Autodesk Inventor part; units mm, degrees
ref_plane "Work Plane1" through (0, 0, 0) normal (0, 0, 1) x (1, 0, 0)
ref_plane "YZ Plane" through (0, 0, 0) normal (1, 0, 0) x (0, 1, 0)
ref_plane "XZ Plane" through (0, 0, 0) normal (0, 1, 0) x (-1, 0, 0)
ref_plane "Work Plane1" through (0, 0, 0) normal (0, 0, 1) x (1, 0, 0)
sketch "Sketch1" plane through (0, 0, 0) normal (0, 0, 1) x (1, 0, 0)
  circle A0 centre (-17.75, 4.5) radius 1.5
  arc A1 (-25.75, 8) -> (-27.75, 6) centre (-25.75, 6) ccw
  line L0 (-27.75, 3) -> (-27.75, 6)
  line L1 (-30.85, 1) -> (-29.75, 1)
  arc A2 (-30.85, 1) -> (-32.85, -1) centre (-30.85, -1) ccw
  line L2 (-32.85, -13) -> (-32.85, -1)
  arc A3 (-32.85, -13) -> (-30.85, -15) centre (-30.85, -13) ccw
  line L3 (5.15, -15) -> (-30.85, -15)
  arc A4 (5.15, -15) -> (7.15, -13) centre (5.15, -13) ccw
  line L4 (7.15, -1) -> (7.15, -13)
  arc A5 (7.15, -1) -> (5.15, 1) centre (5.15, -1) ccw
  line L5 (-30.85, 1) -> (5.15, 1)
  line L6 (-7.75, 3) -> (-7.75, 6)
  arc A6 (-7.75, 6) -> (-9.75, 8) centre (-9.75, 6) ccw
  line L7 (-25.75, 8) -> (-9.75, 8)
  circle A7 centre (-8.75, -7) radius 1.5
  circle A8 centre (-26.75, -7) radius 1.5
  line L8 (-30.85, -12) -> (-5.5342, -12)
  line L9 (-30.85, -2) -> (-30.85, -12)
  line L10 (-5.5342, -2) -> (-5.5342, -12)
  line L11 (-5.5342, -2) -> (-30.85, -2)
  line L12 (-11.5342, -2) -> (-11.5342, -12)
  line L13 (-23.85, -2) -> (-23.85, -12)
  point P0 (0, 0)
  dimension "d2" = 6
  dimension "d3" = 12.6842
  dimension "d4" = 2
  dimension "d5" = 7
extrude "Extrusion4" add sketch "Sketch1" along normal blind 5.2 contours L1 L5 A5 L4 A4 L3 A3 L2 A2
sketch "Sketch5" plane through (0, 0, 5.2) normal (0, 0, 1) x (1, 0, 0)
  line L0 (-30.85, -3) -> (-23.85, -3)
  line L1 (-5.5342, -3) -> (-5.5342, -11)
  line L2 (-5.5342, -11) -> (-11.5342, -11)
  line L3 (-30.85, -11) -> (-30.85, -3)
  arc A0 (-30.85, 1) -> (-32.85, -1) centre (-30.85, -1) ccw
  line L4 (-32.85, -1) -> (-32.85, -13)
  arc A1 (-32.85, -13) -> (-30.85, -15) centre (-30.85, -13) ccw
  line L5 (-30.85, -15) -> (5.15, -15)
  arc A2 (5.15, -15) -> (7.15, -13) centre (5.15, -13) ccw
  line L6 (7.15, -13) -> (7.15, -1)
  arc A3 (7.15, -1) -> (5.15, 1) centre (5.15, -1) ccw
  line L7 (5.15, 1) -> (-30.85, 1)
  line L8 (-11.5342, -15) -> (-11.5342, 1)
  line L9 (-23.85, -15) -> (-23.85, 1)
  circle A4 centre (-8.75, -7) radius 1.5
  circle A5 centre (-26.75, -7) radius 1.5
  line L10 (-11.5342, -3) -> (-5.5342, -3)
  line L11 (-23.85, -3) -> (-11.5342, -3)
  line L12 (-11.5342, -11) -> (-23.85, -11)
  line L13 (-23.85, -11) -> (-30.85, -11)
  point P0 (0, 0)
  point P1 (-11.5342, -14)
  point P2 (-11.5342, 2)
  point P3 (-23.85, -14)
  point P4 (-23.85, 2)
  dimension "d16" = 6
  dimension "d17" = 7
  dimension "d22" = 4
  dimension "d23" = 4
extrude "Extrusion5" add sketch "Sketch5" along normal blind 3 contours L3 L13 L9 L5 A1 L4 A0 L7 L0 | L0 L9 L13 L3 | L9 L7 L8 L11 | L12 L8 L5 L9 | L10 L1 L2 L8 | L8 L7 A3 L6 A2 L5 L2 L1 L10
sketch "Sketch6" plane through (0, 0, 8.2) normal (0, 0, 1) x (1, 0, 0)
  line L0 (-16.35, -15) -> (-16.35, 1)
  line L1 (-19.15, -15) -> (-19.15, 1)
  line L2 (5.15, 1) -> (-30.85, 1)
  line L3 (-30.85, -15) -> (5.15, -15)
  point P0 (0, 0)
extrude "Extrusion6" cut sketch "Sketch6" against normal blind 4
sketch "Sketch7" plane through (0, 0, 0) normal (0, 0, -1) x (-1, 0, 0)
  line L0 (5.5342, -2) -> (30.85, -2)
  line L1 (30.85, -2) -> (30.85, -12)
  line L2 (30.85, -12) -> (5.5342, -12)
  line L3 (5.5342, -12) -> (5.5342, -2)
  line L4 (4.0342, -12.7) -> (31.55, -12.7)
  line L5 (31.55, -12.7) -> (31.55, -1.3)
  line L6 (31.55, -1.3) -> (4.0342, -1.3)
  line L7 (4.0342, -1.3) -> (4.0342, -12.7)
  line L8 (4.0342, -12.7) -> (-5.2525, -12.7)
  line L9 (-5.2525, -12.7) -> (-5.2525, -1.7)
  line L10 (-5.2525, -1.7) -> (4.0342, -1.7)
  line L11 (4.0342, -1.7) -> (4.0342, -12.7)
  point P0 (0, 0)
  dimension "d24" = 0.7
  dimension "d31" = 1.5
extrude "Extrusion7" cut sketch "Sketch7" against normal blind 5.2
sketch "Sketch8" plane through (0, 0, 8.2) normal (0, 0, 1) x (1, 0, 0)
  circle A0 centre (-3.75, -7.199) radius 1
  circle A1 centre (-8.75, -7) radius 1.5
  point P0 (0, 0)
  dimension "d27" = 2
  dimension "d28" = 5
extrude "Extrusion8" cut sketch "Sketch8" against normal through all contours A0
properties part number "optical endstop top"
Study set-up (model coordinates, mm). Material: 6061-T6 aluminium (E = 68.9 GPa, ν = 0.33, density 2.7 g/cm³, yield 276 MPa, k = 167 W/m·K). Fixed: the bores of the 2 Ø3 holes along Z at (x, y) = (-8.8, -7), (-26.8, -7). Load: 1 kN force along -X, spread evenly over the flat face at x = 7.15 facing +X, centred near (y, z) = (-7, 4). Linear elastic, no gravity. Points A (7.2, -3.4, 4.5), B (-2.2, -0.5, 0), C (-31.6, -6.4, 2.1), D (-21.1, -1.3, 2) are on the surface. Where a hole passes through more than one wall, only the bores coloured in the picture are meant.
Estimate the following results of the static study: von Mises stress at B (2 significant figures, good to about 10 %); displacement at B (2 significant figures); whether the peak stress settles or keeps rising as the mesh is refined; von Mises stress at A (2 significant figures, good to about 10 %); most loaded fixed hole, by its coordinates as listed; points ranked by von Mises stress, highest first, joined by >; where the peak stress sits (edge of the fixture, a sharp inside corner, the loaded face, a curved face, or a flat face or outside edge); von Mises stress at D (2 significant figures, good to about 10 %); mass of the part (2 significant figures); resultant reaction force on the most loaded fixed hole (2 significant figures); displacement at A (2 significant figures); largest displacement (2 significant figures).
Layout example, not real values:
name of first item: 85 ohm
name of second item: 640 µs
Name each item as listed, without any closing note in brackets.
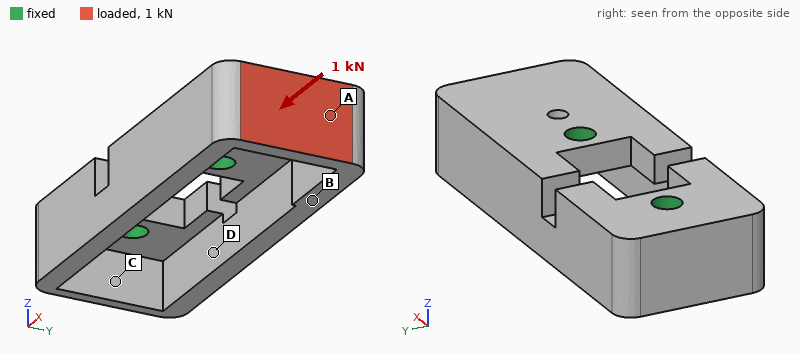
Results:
von Mises stress at B: 35 MPa
displacement at B: 13 µm
whether the peak stress settles or keeps rising as the mesh is refined: keeps rising
von Mises stress at A: 58 MPa
most loaded fixed hole, by its coordinates as listed: (-8.8, -7)
points ranked by von Mises stress, highest first, joined by >: A > B > D > C
where the peak stress sits: edge of the fixture
von Mises stress at D: 15 MPa
mass of the part: 7.1 g
resultant reaction force on the most loaded fixed hole: 750 N
displacement at A: 24 µm
largest displacement: 42 µm
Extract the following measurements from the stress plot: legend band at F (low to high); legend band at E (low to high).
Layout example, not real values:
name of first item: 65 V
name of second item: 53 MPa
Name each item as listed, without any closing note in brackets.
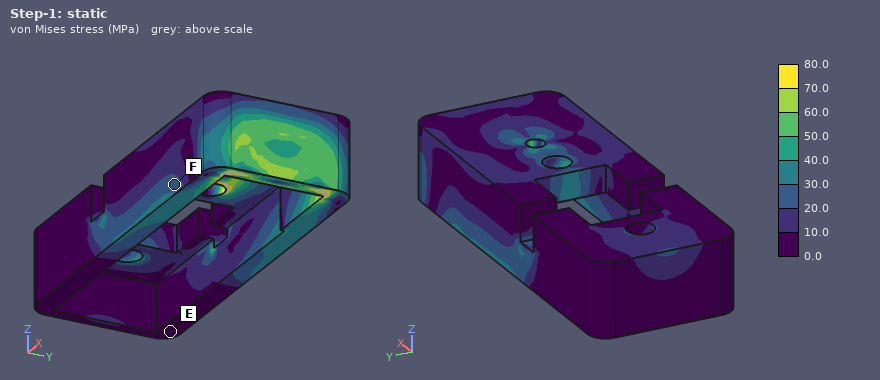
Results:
legend band at F: 20.0 to 30.0 MPa
legend band at E: 0.0 to 10.0 MPa
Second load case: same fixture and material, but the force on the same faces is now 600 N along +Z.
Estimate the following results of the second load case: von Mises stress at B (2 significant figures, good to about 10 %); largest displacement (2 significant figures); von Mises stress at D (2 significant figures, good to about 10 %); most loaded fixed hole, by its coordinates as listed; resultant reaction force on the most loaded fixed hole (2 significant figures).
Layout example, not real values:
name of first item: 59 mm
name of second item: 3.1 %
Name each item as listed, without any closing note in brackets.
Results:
von Mises stress at B: 78 MPa
largest displacement: 0.11 mm
von Mises stress at D: 45 MPa
most loaded fixed hole, by its coordinates as listed: (-8.8, -7)
resultant reaction force on the most loaded fixed hole: 1.1 kN
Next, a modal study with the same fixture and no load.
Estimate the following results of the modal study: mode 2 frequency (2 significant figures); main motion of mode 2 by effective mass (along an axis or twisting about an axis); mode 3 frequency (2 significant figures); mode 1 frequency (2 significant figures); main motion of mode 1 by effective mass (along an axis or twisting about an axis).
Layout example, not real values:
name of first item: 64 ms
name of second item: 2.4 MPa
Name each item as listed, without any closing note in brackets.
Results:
mode 2 frequency: 11 kHz
main motion of mode 2 by effective mass: along Z
mode 3 frequency: 14 kHz
mode 1 frequency: 9900 Hz
main motion of mode 1 by effective mass: along Y
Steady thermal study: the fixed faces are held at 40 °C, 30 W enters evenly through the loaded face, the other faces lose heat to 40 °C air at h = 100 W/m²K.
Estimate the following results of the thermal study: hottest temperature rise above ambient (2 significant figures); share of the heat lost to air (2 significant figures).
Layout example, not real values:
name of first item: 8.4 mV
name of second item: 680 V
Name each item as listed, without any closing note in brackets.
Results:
hottest temperature rise above ambient: 54 K
share of the heat lost to air: 11 %
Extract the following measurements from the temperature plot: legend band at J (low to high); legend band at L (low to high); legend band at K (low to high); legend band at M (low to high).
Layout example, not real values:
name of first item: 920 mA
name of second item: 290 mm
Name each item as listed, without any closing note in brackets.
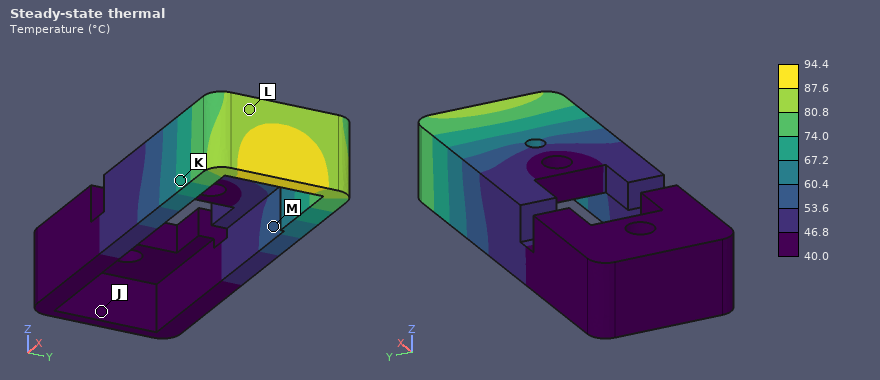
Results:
legend band at J: 40.0 to 46.8 °C
legend band at L: 80.8 to 87.6 °C
legend band at K: 67.2 to 74.0 °C
legend band at M: 53.6 to 60.4 °C
